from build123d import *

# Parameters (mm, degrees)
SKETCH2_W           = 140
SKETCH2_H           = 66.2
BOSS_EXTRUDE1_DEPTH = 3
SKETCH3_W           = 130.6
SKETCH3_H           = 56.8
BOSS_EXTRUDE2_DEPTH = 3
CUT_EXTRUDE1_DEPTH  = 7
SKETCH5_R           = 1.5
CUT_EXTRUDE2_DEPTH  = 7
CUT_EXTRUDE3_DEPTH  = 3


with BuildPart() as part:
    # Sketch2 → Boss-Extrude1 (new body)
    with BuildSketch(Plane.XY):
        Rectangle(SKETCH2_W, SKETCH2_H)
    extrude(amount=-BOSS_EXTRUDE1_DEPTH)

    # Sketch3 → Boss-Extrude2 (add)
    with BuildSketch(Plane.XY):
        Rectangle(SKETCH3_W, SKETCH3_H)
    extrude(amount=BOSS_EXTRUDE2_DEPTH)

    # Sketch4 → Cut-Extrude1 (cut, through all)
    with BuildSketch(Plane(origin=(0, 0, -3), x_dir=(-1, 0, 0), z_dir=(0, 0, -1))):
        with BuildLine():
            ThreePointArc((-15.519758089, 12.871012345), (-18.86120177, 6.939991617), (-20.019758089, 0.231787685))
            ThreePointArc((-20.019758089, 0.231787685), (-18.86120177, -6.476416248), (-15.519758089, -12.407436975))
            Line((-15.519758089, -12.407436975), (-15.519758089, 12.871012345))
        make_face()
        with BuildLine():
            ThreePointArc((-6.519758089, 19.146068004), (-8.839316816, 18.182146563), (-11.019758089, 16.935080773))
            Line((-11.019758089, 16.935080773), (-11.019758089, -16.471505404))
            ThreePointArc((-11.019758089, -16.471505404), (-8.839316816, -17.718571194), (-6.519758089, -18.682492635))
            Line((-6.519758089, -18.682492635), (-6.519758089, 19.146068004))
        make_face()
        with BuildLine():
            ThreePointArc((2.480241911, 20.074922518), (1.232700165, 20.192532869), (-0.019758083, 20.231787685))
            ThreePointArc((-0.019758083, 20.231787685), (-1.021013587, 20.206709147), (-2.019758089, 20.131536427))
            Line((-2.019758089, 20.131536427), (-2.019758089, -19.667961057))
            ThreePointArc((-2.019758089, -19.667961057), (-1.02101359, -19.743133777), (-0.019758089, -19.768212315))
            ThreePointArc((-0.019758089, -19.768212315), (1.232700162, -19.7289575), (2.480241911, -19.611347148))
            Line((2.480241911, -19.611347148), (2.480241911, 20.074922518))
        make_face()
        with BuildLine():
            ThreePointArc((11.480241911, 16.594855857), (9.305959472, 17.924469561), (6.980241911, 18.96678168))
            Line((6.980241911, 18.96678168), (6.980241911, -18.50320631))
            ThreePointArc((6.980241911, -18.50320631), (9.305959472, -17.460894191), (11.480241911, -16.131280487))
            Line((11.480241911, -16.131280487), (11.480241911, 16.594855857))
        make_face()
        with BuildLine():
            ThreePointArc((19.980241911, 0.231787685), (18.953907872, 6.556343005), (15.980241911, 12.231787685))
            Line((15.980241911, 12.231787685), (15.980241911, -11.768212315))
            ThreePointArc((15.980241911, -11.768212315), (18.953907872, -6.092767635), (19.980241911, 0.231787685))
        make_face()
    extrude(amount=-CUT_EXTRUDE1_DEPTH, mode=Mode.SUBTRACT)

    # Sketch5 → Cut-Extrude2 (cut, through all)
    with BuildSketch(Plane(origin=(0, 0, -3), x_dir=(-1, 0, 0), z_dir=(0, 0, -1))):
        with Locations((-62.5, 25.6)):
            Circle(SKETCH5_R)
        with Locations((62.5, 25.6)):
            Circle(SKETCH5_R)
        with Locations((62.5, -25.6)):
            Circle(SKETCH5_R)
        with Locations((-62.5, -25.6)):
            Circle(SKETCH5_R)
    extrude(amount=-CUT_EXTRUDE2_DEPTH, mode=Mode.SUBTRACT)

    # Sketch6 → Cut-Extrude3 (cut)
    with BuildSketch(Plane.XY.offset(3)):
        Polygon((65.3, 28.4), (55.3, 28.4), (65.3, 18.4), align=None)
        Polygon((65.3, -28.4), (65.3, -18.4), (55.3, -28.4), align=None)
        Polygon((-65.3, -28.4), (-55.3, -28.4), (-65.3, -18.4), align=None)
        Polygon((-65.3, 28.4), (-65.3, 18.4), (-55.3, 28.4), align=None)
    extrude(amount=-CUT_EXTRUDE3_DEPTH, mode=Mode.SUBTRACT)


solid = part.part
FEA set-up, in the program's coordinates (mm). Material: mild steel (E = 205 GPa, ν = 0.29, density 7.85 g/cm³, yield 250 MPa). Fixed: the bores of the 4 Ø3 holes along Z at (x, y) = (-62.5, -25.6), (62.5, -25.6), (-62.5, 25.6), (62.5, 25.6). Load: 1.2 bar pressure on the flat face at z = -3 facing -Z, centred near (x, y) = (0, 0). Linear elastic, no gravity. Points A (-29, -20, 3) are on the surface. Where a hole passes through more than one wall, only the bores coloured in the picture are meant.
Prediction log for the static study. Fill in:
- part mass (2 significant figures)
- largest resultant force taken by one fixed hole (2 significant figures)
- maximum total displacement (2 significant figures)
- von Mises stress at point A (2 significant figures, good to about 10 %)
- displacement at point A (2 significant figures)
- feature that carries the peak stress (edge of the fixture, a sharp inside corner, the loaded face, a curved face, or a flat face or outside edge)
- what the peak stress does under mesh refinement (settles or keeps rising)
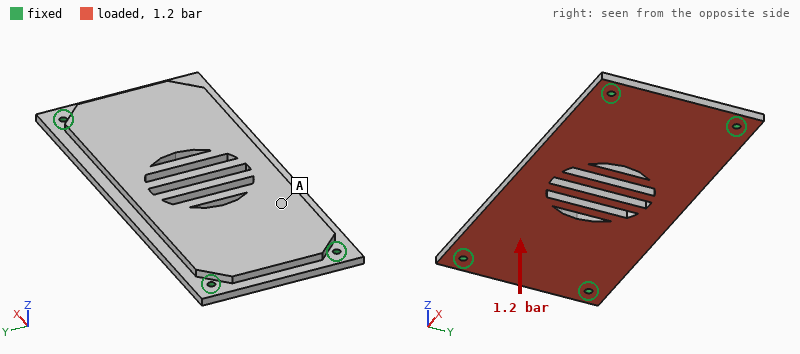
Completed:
360 g
560 N
75 µm
15 MPa
48 µm
edge of the fixture
keeps rising
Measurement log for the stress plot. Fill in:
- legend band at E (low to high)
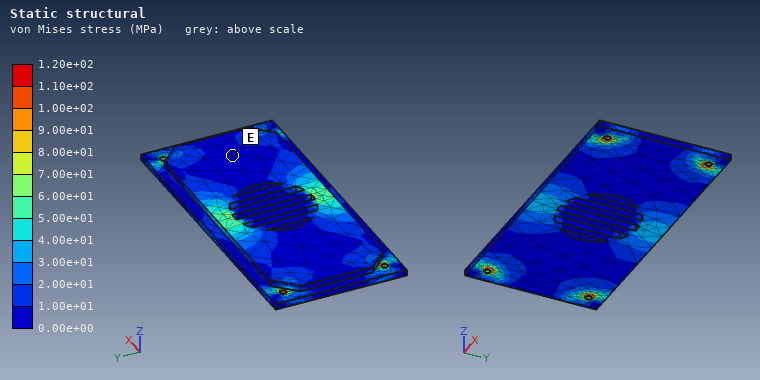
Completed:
0.00e+00 to 1.00e+01 MPa
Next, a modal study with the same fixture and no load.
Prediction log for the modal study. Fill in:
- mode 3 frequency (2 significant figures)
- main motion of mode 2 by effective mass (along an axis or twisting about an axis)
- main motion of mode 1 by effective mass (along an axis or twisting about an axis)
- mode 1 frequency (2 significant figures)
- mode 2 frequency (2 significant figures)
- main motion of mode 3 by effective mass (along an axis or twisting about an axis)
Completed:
3500 Hz
twisting about X
along Z
1100 Hz
2700 Hz
twisting about Y
